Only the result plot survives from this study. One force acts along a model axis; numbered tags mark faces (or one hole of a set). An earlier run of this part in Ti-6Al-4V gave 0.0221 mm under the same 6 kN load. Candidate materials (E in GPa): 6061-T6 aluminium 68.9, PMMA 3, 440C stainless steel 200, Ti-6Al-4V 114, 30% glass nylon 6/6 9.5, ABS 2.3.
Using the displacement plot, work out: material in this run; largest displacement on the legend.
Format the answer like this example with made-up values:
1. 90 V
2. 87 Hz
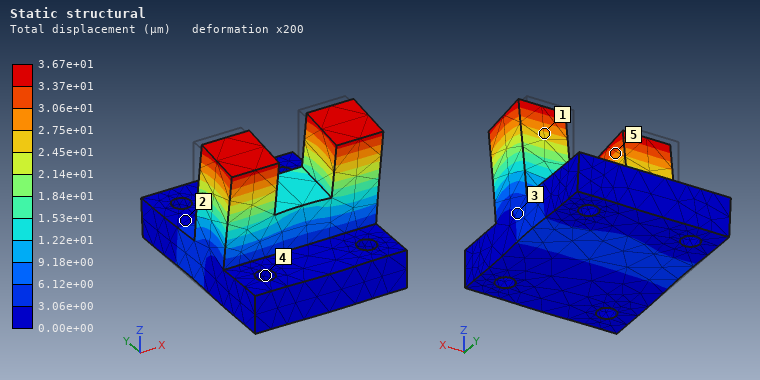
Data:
1. 6061-T6 aluminium
2. 3.67e+01 µm
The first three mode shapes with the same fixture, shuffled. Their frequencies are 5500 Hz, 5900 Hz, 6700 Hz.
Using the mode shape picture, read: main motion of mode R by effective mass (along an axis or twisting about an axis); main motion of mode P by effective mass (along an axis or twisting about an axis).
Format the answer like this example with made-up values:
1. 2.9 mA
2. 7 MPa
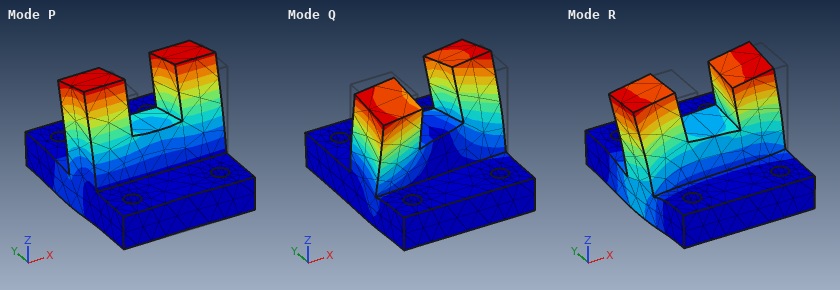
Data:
1. along X
2. along Y
